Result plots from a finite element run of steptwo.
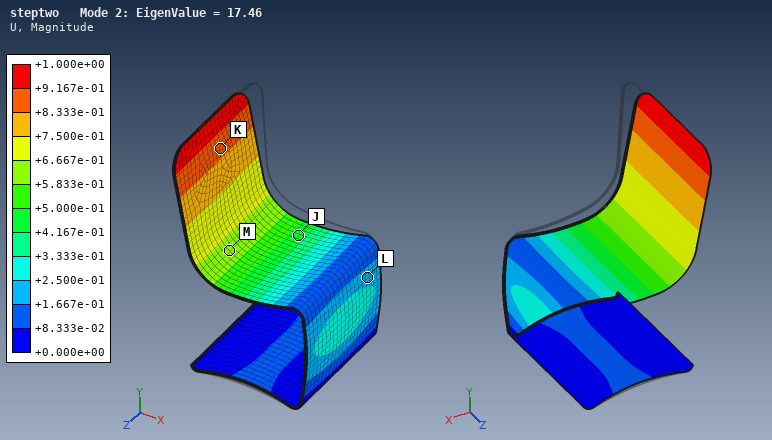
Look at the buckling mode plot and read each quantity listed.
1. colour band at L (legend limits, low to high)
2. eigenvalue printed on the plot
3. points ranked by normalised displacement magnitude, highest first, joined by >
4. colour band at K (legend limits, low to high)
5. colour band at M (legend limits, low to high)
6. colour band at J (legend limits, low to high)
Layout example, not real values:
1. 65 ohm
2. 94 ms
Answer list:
1. +1.667e-01 to +2.500e-01
2. 17.46
3. K > M > J > L
4. +8.333e-01 to +9.167e-01
5. +5.833e-01 to +6.667e-01
6. +4.167e-01 to +5.000e-01
